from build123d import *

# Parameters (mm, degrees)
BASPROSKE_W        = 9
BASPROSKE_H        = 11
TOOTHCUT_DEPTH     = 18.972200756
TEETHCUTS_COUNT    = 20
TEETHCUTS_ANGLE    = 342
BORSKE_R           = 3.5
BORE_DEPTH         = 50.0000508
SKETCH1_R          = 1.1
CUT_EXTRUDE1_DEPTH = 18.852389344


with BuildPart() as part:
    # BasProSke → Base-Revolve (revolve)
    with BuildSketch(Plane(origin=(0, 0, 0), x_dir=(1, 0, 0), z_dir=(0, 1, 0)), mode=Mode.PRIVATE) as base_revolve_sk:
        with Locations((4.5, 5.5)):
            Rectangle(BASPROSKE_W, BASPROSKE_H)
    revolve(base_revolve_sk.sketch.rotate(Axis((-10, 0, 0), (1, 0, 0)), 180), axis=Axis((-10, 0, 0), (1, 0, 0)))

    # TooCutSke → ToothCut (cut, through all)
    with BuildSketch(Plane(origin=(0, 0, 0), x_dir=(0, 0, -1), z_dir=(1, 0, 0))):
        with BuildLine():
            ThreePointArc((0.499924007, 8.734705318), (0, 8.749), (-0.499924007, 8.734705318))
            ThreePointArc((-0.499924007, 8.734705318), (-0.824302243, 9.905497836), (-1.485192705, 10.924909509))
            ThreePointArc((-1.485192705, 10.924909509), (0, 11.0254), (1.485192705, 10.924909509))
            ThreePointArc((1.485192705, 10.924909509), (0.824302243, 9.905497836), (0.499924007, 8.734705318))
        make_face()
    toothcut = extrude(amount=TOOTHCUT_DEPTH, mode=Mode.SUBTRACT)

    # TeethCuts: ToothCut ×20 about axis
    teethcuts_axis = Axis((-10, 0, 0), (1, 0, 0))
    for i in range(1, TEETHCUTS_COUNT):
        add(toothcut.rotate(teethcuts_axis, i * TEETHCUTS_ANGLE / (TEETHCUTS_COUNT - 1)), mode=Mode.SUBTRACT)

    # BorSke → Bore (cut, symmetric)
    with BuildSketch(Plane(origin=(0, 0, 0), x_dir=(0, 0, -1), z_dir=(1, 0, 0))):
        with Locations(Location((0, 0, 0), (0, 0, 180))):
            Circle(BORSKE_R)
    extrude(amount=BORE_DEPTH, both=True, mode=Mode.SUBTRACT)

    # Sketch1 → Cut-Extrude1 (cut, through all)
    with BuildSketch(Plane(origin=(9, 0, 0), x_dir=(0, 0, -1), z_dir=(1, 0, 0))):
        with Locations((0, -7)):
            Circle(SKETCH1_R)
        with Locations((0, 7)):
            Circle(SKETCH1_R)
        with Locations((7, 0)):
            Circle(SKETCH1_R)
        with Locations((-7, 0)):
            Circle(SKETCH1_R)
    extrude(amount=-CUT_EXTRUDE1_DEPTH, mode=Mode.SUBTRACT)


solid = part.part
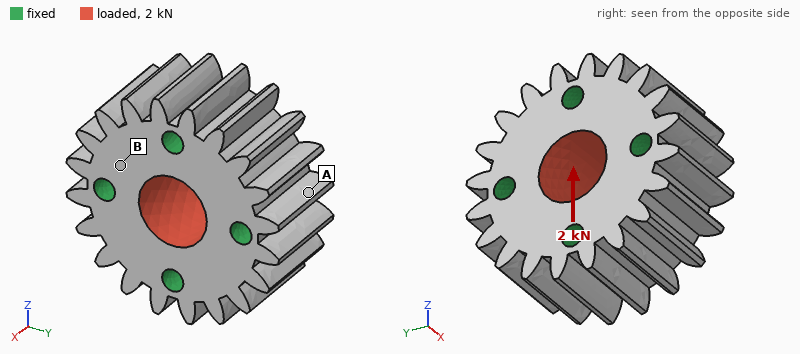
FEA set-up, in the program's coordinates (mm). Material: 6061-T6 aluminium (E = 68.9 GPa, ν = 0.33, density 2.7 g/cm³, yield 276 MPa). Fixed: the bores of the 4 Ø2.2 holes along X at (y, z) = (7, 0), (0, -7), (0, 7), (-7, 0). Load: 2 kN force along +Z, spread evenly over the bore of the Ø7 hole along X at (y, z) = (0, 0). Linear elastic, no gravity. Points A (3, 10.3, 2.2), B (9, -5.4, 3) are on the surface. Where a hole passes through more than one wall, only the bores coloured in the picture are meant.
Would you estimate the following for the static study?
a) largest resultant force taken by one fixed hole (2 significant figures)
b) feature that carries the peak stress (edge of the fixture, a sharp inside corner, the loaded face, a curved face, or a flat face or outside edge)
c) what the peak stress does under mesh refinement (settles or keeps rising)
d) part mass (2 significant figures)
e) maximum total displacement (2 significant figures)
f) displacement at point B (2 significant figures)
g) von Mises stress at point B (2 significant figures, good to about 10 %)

580 N
edge of the fixture
keeps rising
6.1 g
1.00 µm
0.51 µm
6.4 MPa
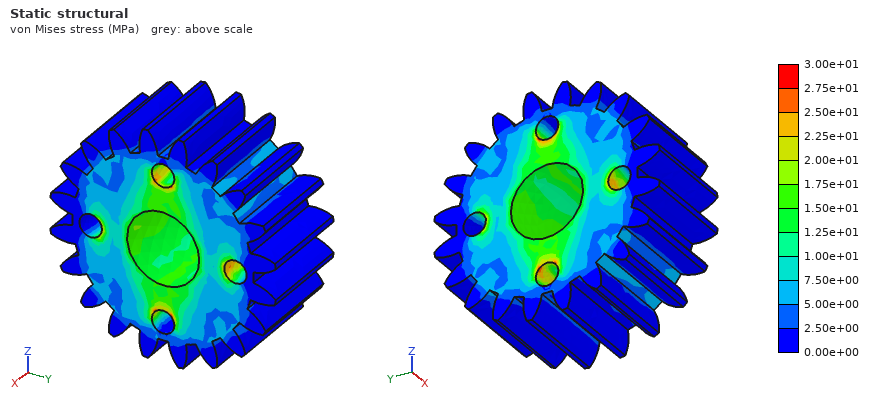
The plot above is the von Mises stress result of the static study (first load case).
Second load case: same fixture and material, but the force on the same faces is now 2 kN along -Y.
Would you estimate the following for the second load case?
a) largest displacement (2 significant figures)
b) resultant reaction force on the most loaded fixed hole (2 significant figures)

1.00 µm
580 N
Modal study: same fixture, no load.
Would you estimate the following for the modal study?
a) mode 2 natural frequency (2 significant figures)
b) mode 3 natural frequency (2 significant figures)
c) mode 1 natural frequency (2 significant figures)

110 kHz
110 kHz
100 kHz
